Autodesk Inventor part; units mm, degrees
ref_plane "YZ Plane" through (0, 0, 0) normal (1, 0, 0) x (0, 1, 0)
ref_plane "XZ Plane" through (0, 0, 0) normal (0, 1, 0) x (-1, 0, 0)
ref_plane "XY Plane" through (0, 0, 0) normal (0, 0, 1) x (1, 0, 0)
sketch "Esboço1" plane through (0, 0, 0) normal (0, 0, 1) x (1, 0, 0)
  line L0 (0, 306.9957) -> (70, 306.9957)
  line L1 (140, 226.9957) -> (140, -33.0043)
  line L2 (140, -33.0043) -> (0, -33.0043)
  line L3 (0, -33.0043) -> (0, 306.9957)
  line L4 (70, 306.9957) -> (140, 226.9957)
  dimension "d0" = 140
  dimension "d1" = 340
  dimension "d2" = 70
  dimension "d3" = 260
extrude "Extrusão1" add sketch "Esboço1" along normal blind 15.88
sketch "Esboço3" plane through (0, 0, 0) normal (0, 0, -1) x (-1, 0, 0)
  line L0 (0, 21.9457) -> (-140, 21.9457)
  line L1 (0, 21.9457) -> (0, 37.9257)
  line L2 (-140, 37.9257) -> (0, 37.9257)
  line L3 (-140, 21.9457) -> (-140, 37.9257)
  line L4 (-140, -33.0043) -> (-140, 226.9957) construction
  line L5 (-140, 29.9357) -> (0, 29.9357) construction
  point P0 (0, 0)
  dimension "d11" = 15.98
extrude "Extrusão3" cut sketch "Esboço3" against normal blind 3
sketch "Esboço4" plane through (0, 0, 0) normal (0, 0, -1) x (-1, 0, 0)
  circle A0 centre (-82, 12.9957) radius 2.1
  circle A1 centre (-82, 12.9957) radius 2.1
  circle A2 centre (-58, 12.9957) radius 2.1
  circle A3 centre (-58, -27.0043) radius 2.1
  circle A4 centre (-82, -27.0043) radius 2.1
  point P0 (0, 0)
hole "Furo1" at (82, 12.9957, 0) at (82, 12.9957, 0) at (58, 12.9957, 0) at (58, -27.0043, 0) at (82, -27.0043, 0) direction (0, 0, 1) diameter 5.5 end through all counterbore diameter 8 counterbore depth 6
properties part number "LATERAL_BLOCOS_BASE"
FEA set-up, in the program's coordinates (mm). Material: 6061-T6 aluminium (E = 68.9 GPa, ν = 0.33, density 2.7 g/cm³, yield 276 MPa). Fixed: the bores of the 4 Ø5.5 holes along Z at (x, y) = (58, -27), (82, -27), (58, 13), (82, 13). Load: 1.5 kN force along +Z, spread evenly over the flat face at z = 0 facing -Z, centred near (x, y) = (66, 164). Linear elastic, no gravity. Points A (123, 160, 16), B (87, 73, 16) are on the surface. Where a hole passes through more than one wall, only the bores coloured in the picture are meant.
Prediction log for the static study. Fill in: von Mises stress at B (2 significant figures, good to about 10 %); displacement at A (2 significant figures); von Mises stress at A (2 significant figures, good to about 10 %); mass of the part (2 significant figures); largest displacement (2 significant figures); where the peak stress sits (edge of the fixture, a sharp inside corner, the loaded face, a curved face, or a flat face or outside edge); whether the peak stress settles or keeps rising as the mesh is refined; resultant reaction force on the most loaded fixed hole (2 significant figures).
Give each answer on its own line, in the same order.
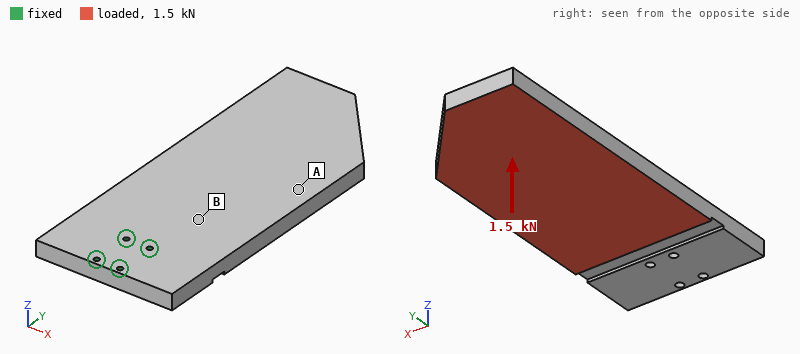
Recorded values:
22 MPa
0.81 mm
8.6 MPa
1.9 kg
2.1 mm
edge of the fixture
keeps rising
3.3 kN
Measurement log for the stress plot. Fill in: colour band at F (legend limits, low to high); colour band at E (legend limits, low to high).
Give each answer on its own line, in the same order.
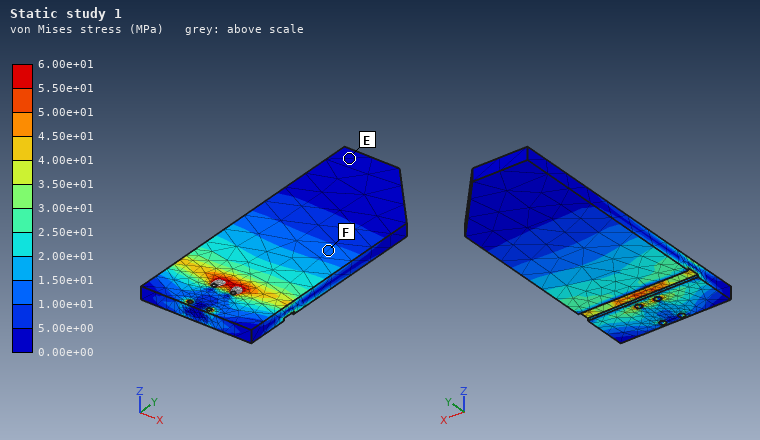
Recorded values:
1.00e+01 to 1.50e+01 MPa
0.00e+00 to 5.00e+00 MPa
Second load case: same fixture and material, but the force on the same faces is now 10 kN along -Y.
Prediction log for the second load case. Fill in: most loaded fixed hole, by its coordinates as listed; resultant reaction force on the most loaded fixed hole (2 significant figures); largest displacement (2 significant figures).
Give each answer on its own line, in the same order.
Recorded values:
(58, 13)
3.7 kN
1.0 mm
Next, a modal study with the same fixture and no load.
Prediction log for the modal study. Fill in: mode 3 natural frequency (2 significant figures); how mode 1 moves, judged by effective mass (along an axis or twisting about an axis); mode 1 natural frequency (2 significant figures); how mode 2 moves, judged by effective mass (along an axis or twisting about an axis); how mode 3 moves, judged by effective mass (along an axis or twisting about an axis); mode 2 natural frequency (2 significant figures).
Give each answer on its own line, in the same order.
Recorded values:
720 Hz
along Z
140 Hz
twisting about Y
along X
600 Hz
